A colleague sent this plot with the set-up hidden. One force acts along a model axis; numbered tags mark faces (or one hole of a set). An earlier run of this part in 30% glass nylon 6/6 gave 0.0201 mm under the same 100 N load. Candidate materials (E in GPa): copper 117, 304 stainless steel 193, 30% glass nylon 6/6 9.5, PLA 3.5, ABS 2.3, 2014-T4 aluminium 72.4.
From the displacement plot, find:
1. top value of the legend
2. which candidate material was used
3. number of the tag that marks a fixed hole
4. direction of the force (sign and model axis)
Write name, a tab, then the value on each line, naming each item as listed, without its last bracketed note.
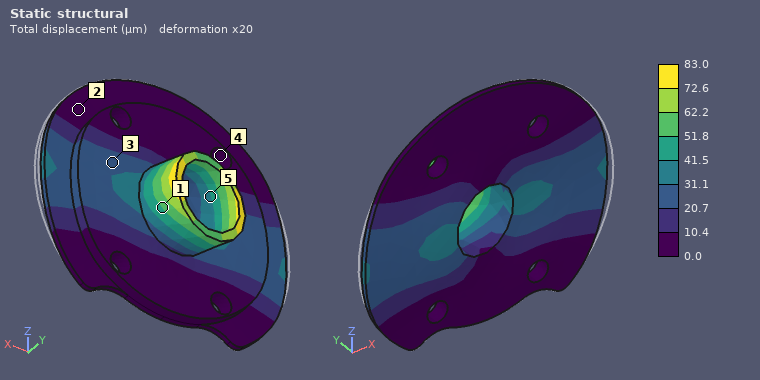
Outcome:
top value of the legend	83.0 µm
which candidate material was used	ABS
number of the tag that marks a fixed hole	4
direction of the force	-X
